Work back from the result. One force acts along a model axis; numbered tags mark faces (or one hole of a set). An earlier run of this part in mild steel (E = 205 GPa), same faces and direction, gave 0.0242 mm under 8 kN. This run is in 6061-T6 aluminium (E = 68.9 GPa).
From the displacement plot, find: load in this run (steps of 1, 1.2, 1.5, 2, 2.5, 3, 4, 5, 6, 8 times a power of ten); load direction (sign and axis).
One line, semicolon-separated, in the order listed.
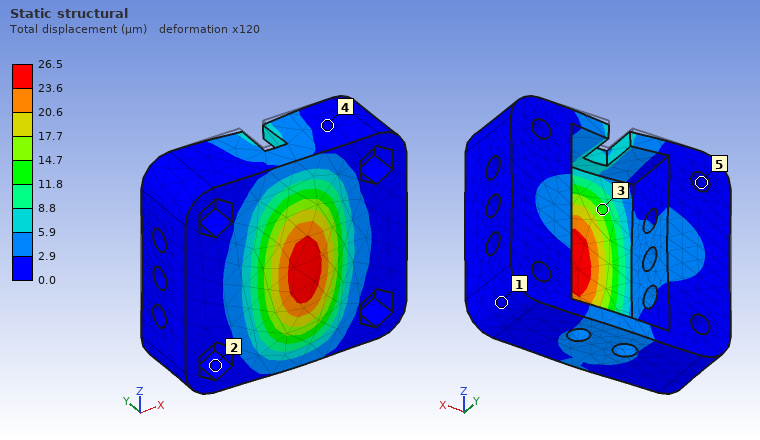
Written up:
3 kN; -Y
